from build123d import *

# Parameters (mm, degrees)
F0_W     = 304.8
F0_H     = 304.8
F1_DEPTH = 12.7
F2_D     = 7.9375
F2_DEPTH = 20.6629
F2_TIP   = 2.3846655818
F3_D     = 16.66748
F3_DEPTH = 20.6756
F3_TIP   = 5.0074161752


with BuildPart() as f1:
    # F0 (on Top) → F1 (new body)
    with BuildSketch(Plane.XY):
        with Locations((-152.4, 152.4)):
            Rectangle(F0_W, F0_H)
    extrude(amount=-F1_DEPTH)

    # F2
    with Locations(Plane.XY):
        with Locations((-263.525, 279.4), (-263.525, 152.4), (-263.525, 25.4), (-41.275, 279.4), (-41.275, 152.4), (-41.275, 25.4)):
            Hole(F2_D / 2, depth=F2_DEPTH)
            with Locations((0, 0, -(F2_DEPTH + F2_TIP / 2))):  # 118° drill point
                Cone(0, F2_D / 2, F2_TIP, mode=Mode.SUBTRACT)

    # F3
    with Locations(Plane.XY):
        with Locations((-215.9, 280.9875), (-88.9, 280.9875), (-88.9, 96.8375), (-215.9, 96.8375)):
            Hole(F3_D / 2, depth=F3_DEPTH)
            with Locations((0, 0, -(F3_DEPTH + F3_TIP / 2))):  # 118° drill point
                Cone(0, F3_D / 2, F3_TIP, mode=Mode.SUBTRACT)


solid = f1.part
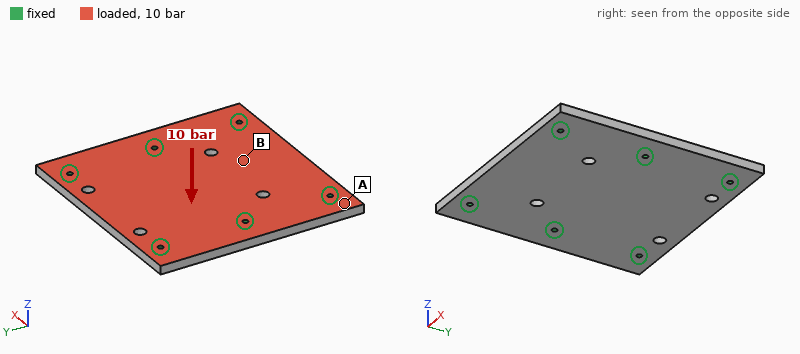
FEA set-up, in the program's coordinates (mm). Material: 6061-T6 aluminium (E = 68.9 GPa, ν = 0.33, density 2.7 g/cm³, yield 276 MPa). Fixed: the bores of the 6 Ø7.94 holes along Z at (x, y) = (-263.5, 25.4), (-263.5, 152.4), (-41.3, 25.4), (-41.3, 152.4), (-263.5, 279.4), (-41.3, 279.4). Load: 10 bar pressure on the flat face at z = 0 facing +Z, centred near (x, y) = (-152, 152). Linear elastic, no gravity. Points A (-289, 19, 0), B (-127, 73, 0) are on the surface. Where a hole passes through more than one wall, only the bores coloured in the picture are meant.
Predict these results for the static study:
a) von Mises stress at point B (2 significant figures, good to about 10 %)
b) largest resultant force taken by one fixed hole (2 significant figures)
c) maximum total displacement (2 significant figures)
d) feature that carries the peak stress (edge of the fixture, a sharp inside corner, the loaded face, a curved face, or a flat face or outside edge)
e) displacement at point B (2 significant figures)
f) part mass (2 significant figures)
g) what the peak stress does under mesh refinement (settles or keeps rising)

67 MPa
20 kN
0.79 mm
edge of the fixture
0.71 mm
3.1 kg
keeps rising
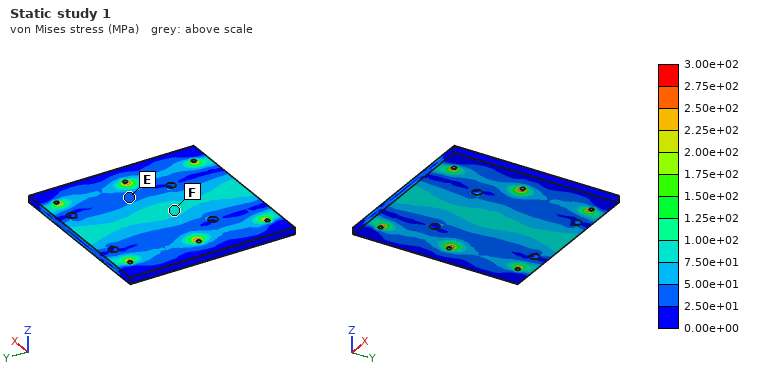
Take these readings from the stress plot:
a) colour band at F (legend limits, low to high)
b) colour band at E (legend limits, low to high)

7.50e+01 to 1.00e+02 MPa
2.50e+01 to 5.00e+01 MPa
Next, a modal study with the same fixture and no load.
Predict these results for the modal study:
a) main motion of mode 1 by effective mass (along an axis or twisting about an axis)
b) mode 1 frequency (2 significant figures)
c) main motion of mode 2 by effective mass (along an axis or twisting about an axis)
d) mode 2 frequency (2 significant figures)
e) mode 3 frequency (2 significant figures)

along Z
1100 Hz
twisting about X
1300 Hz
1900 Hz
